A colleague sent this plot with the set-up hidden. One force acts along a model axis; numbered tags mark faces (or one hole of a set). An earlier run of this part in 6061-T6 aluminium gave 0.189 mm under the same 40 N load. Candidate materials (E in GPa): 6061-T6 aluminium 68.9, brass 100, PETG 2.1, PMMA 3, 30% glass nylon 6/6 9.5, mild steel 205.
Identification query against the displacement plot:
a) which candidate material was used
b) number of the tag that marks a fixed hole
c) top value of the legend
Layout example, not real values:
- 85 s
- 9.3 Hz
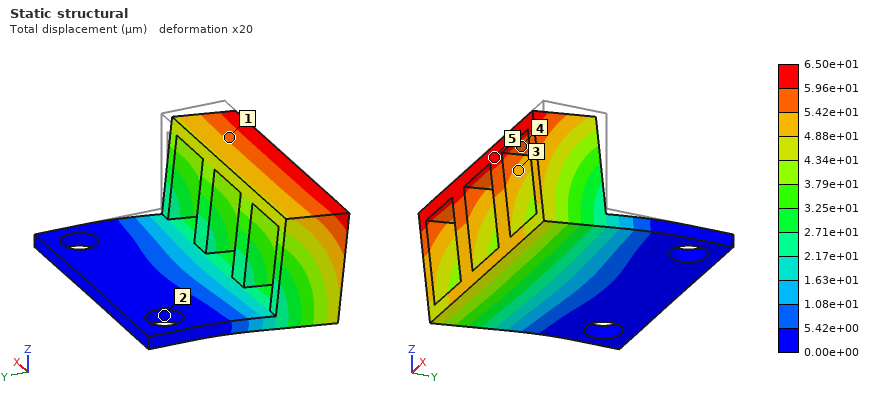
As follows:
- mild steel
- 2
- 6.50e+01 µm
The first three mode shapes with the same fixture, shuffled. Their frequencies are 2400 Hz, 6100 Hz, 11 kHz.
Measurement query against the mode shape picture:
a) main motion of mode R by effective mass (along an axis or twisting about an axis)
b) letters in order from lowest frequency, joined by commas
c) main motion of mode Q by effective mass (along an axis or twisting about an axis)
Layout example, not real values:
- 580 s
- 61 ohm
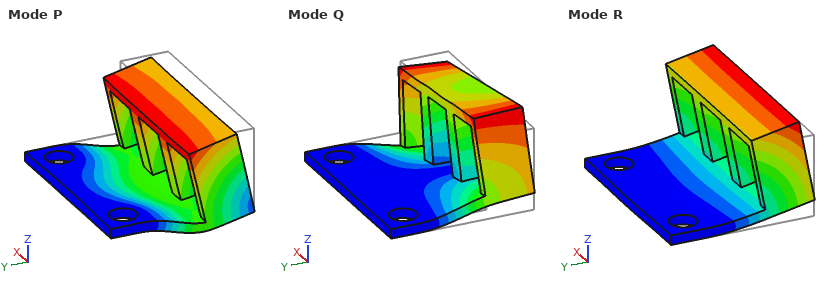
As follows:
- along Z
- R, Q, P
- along X
